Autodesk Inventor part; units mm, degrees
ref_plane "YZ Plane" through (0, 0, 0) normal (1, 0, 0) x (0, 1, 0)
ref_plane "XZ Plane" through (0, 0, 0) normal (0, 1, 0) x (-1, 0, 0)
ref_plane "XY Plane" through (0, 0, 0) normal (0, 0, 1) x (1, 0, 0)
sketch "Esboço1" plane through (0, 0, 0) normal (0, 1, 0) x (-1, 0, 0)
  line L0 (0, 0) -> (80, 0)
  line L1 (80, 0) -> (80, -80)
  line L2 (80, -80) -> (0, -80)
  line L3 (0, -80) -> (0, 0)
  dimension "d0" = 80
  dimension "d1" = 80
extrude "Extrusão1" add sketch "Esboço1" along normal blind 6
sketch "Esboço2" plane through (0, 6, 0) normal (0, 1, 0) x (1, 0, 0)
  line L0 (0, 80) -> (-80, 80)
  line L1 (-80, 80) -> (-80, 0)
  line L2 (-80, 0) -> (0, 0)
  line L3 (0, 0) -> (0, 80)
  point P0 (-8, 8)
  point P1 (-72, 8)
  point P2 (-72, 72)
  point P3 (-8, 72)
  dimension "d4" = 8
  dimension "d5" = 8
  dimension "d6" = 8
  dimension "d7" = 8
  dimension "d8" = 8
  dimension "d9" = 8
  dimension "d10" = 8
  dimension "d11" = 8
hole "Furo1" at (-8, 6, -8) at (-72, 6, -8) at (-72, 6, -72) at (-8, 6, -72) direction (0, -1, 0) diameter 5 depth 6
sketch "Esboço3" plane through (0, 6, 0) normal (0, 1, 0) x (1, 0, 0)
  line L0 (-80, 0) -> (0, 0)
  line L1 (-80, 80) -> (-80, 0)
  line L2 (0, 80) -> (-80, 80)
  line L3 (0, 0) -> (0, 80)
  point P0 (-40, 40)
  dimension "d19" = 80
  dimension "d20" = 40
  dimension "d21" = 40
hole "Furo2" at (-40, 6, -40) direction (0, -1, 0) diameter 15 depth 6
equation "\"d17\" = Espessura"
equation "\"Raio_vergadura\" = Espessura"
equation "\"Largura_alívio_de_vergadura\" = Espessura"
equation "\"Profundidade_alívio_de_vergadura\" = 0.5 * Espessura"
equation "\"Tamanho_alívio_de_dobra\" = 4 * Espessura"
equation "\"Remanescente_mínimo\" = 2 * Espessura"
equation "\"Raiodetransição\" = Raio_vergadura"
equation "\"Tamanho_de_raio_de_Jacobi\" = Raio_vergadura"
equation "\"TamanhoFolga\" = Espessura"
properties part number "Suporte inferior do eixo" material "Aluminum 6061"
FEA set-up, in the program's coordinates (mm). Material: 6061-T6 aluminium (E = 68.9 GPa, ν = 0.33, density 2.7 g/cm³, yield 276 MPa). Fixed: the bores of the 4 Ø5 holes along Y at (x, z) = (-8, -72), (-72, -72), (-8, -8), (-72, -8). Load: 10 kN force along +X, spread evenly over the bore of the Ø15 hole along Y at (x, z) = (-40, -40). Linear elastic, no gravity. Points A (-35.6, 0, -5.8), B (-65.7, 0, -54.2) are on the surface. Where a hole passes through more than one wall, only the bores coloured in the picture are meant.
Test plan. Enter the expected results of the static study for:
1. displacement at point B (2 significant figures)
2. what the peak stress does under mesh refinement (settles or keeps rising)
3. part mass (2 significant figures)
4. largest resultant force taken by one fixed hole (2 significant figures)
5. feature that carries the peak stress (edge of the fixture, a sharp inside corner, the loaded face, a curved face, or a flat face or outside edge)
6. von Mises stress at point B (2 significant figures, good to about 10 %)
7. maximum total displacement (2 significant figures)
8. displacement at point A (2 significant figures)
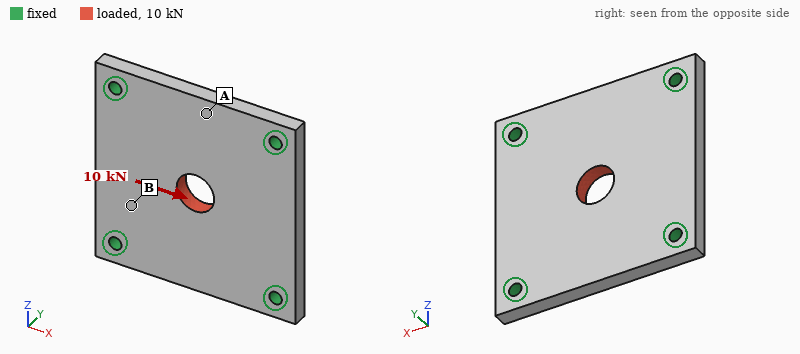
11 µm
keeps rising
100 g
2.8 kN
edge of the fixture
19 MPa
19 µm
4.6 µm
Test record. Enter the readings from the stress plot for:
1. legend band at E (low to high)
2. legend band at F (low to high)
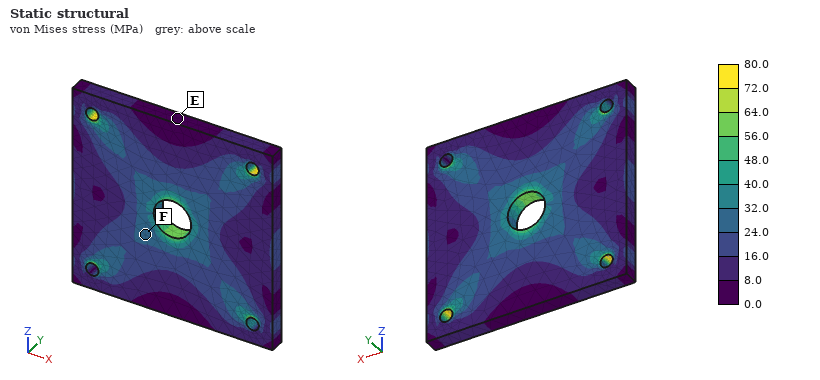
0.0 to 8.0 MPa
24.0 to 32.0 MPa
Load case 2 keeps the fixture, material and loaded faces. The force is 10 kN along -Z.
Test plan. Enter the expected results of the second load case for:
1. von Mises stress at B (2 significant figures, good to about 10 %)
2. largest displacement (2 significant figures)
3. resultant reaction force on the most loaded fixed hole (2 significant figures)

18 MPa
19 µm
2.8 kN
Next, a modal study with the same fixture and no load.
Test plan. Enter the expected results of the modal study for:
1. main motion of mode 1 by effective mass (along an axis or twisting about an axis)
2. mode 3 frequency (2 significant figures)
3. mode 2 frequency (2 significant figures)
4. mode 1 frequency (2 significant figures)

along Y
8000 Hz
8000 Hz
5000 Hz
